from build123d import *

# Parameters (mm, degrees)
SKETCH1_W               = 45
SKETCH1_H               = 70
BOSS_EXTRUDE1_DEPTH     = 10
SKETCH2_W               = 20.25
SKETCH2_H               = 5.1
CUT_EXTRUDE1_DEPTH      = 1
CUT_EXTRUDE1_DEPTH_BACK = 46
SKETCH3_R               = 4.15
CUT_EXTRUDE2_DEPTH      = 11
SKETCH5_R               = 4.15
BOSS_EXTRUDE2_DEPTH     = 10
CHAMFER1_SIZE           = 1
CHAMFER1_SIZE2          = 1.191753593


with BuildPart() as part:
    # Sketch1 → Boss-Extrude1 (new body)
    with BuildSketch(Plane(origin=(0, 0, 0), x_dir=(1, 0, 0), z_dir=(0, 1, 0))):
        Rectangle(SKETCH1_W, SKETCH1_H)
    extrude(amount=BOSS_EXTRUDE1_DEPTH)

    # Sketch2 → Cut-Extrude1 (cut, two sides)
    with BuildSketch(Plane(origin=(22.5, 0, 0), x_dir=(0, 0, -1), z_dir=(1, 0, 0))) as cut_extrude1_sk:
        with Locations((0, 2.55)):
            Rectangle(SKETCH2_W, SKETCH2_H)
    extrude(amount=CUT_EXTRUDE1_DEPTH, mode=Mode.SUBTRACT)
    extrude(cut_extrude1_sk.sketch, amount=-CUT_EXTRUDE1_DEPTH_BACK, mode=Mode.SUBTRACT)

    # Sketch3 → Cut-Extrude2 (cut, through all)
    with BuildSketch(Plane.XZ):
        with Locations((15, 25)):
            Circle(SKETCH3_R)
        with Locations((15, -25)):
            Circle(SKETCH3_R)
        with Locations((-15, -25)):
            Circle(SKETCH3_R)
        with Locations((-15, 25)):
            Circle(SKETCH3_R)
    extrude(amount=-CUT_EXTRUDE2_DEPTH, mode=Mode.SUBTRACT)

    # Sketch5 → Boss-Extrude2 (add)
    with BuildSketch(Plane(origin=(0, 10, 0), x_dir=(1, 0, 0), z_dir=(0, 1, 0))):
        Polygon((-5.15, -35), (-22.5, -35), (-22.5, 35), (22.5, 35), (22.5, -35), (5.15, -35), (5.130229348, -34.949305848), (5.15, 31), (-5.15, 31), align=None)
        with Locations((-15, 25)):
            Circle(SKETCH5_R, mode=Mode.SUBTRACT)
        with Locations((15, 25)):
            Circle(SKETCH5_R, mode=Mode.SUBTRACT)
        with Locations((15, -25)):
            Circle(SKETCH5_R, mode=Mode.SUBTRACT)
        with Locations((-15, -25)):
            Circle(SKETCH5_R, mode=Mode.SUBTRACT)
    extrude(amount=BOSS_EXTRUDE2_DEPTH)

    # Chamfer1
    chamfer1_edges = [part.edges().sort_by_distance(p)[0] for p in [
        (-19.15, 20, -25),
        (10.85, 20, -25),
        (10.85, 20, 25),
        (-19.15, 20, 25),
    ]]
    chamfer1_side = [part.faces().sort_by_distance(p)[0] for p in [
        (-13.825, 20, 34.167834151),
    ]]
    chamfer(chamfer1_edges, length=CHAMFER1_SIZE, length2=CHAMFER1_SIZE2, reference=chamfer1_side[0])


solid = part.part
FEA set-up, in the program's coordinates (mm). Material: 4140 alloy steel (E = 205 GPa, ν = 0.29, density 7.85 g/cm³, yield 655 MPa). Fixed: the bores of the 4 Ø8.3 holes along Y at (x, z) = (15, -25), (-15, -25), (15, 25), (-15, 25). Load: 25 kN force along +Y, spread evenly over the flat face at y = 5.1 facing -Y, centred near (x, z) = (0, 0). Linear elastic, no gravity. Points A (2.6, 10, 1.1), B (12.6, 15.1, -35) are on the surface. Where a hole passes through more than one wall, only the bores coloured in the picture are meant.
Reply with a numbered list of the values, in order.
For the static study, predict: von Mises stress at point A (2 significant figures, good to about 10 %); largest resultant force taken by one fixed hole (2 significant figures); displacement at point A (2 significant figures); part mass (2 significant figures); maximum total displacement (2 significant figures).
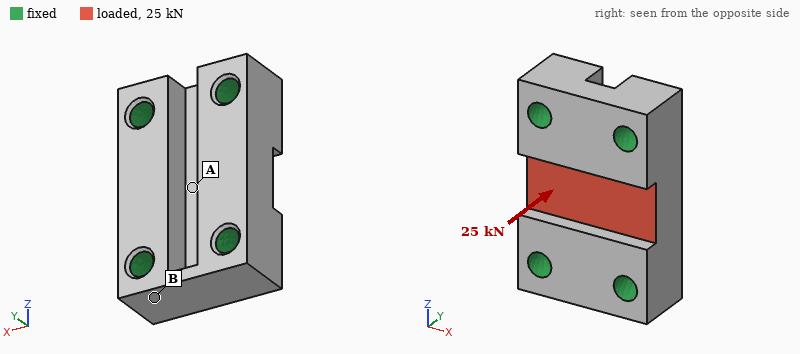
1. 47 MPa
2. 6.3 kN
3. 11 µm
4. 370 g
5. 12 µm
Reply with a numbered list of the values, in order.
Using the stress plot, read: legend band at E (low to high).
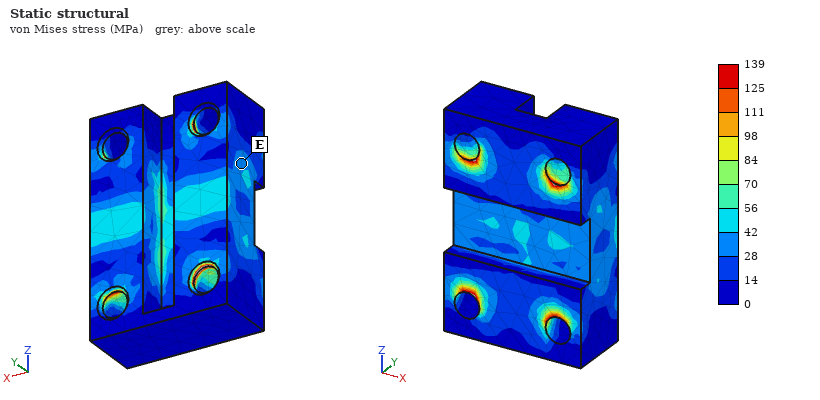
1. 28 to 42 MPa
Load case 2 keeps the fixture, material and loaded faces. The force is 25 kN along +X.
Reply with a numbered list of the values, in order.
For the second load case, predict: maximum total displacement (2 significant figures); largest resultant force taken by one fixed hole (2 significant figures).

1. 11 µm
2. 7.1 kN
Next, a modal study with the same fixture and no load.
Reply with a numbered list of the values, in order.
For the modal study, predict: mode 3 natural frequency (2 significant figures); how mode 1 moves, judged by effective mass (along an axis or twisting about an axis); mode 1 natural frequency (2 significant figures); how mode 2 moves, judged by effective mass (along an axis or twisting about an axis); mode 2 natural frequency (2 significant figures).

1. 31 kHz
2. along Y
3. 27 kHz
4. along X
5. 28 kHz
